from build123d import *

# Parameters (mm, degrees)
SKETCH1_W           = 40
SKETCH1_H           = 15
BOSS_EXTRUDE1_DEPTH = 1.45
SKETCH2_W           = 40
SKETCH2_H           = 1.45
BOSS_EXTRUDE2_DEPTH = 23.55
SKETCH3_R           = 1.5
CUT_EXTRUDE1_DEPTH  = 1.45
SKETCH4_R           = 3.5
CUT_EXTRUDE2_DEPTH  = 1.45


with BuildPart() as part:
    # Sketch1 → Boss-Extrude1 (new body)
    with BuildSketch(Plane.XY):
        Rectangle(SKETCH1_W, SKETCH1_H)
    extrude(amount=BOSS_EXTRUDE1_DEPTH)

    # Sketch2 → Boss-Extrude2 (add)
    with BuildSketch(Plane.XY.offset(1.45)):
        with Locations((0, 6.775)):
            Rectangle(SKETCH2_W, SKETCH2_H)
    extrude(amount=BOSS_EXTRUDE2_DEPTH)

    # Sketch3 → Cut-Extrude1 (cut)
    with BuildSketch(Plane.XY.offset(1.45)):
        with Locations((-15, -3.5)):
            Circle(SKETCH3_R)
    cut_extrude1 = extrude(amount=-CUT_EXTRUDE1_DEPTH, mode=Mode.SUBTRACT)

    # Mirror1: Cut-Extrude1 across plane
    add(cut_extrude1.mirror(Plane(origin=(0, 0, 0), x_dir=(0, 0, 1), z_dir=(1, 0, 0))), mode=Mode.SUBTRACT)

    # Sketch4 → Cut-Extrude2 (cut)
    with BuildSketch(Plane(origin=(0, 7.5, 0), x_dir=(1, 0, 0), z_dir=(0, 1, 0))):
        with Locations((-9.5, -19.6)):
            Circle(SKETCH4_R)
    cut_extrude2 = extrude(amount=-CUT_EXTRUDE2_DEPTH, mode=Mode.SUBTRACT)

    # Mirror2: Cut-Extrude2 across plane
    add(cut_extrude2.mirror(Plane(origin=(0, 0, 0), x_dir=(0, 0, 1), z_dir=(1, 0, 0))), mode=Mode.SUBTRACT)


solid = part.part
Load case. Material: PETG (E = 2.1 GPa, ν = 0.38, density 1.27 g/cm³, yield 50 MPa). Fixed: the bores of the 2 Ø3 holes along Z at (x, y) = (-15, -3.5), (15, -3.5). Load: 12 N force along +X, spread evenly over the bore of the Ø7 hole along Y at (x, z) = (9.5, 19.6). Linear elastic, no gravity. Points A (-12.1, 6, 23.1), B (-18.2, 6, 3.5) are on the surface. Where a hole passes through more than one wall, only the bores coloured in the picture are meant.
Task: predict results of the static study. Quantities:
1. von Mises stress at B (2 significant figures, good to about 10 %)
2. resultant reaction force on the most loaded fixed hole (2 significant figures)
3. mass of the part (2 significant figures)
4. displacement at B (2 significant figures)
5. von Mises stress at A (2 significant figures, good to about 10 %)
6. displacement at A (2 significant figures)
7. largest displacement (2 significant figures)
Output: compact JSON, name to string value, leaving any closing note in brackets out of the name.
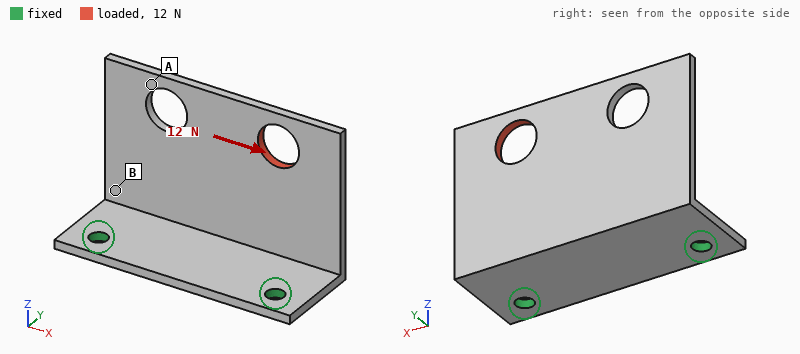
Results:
{"von Mises stress at B": "4.1 MPa", "resultant reaction force on the most loaded fixed hole": "10 N", "mass of the part": "2.7 g", "displacement at B": "0.21 mm", "von Mises stress at A": "1.2 MPa", "displacement at A": "0.37 mm", "largest displacement": "0.50 mm"}
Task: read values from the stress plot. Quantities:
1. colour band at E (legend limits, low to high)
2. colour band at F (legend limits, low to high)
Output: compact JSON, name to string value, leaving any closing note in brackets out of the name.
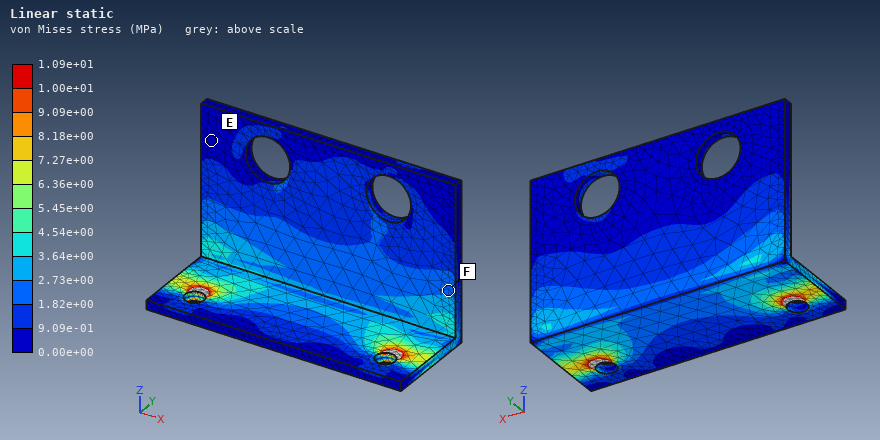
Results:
{"colour band at E": "0.00e+00 to 9.09e-01 MPa", "colour band at F": "1.82e+00 to 2.73e+00 MPa"}
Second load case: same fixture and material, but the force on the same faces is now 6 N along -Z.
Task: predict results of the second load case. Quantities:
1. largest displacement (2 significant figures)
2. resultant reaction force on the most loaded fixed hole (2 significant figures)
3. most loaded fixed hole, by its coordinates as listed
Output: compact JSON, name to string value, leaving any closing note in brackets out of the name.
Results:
{"largest displacement": "0.51 mm", "resultant reaction force on the most loaded fixed hole": "4.9 N", "most loaded fixed hole, by its coordinates as listed": "(15, -3.5)"}
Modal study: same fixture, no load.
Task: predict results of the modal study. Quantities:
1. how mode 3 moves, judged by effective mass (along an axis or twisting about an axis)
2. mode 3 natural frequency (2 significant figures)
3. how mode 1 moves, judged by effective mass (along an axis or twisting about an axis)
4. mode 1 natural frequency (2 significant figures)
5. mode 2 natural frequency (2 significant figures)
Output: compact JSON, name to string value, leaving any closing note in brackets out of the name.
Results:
{"how mode 3 moves, judged by effective mass": "along X", "mode 3 natural frequency": "1100 Hz", "how mode 1 moves, judged by effective mass": "along Y", "mode 1 natural frequency": "330 Hz", "mode 2 natural frequency": "670 Hz"}
